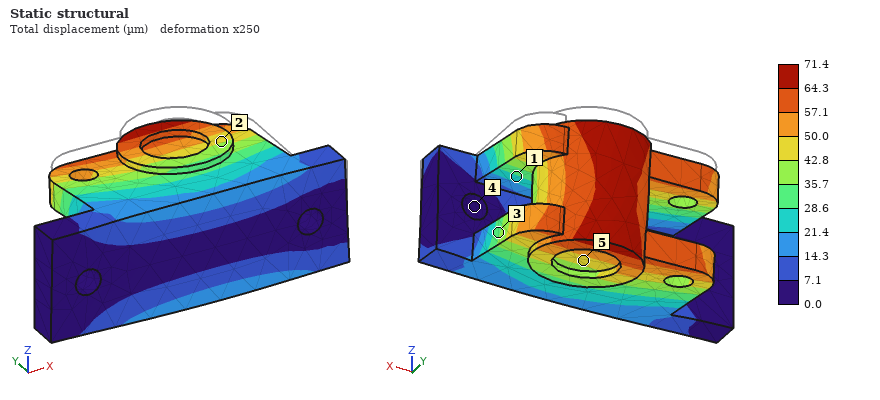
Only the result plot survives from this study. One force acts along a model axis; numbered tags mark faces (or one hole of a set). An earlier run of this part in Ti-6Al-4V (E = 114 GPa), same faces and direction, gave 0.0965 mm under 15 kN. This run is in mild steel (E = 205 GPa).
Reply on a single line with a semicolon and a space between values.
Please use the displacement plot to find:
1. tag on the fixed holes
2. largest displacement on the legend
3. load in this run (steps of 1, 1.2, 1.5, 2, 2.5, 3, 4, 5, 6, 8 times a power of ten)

4; 71.4 µm; 20 kN
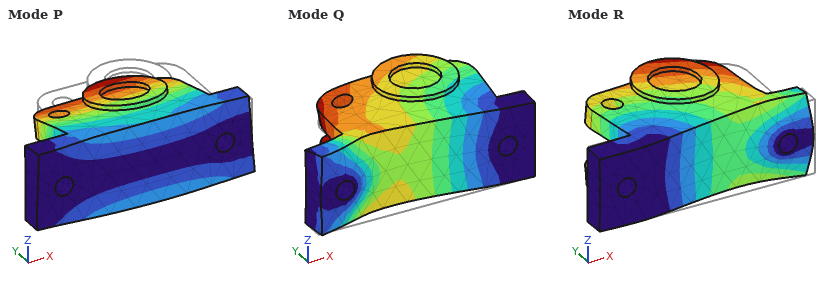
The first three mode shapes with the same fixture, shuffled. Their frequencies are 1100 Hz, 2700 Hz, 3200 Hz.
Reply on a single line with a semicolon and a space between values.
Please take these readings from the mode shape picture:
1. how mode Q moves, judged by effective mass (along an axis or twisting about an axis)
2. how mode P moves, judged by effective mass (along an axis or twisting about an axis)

along Y; along Z
